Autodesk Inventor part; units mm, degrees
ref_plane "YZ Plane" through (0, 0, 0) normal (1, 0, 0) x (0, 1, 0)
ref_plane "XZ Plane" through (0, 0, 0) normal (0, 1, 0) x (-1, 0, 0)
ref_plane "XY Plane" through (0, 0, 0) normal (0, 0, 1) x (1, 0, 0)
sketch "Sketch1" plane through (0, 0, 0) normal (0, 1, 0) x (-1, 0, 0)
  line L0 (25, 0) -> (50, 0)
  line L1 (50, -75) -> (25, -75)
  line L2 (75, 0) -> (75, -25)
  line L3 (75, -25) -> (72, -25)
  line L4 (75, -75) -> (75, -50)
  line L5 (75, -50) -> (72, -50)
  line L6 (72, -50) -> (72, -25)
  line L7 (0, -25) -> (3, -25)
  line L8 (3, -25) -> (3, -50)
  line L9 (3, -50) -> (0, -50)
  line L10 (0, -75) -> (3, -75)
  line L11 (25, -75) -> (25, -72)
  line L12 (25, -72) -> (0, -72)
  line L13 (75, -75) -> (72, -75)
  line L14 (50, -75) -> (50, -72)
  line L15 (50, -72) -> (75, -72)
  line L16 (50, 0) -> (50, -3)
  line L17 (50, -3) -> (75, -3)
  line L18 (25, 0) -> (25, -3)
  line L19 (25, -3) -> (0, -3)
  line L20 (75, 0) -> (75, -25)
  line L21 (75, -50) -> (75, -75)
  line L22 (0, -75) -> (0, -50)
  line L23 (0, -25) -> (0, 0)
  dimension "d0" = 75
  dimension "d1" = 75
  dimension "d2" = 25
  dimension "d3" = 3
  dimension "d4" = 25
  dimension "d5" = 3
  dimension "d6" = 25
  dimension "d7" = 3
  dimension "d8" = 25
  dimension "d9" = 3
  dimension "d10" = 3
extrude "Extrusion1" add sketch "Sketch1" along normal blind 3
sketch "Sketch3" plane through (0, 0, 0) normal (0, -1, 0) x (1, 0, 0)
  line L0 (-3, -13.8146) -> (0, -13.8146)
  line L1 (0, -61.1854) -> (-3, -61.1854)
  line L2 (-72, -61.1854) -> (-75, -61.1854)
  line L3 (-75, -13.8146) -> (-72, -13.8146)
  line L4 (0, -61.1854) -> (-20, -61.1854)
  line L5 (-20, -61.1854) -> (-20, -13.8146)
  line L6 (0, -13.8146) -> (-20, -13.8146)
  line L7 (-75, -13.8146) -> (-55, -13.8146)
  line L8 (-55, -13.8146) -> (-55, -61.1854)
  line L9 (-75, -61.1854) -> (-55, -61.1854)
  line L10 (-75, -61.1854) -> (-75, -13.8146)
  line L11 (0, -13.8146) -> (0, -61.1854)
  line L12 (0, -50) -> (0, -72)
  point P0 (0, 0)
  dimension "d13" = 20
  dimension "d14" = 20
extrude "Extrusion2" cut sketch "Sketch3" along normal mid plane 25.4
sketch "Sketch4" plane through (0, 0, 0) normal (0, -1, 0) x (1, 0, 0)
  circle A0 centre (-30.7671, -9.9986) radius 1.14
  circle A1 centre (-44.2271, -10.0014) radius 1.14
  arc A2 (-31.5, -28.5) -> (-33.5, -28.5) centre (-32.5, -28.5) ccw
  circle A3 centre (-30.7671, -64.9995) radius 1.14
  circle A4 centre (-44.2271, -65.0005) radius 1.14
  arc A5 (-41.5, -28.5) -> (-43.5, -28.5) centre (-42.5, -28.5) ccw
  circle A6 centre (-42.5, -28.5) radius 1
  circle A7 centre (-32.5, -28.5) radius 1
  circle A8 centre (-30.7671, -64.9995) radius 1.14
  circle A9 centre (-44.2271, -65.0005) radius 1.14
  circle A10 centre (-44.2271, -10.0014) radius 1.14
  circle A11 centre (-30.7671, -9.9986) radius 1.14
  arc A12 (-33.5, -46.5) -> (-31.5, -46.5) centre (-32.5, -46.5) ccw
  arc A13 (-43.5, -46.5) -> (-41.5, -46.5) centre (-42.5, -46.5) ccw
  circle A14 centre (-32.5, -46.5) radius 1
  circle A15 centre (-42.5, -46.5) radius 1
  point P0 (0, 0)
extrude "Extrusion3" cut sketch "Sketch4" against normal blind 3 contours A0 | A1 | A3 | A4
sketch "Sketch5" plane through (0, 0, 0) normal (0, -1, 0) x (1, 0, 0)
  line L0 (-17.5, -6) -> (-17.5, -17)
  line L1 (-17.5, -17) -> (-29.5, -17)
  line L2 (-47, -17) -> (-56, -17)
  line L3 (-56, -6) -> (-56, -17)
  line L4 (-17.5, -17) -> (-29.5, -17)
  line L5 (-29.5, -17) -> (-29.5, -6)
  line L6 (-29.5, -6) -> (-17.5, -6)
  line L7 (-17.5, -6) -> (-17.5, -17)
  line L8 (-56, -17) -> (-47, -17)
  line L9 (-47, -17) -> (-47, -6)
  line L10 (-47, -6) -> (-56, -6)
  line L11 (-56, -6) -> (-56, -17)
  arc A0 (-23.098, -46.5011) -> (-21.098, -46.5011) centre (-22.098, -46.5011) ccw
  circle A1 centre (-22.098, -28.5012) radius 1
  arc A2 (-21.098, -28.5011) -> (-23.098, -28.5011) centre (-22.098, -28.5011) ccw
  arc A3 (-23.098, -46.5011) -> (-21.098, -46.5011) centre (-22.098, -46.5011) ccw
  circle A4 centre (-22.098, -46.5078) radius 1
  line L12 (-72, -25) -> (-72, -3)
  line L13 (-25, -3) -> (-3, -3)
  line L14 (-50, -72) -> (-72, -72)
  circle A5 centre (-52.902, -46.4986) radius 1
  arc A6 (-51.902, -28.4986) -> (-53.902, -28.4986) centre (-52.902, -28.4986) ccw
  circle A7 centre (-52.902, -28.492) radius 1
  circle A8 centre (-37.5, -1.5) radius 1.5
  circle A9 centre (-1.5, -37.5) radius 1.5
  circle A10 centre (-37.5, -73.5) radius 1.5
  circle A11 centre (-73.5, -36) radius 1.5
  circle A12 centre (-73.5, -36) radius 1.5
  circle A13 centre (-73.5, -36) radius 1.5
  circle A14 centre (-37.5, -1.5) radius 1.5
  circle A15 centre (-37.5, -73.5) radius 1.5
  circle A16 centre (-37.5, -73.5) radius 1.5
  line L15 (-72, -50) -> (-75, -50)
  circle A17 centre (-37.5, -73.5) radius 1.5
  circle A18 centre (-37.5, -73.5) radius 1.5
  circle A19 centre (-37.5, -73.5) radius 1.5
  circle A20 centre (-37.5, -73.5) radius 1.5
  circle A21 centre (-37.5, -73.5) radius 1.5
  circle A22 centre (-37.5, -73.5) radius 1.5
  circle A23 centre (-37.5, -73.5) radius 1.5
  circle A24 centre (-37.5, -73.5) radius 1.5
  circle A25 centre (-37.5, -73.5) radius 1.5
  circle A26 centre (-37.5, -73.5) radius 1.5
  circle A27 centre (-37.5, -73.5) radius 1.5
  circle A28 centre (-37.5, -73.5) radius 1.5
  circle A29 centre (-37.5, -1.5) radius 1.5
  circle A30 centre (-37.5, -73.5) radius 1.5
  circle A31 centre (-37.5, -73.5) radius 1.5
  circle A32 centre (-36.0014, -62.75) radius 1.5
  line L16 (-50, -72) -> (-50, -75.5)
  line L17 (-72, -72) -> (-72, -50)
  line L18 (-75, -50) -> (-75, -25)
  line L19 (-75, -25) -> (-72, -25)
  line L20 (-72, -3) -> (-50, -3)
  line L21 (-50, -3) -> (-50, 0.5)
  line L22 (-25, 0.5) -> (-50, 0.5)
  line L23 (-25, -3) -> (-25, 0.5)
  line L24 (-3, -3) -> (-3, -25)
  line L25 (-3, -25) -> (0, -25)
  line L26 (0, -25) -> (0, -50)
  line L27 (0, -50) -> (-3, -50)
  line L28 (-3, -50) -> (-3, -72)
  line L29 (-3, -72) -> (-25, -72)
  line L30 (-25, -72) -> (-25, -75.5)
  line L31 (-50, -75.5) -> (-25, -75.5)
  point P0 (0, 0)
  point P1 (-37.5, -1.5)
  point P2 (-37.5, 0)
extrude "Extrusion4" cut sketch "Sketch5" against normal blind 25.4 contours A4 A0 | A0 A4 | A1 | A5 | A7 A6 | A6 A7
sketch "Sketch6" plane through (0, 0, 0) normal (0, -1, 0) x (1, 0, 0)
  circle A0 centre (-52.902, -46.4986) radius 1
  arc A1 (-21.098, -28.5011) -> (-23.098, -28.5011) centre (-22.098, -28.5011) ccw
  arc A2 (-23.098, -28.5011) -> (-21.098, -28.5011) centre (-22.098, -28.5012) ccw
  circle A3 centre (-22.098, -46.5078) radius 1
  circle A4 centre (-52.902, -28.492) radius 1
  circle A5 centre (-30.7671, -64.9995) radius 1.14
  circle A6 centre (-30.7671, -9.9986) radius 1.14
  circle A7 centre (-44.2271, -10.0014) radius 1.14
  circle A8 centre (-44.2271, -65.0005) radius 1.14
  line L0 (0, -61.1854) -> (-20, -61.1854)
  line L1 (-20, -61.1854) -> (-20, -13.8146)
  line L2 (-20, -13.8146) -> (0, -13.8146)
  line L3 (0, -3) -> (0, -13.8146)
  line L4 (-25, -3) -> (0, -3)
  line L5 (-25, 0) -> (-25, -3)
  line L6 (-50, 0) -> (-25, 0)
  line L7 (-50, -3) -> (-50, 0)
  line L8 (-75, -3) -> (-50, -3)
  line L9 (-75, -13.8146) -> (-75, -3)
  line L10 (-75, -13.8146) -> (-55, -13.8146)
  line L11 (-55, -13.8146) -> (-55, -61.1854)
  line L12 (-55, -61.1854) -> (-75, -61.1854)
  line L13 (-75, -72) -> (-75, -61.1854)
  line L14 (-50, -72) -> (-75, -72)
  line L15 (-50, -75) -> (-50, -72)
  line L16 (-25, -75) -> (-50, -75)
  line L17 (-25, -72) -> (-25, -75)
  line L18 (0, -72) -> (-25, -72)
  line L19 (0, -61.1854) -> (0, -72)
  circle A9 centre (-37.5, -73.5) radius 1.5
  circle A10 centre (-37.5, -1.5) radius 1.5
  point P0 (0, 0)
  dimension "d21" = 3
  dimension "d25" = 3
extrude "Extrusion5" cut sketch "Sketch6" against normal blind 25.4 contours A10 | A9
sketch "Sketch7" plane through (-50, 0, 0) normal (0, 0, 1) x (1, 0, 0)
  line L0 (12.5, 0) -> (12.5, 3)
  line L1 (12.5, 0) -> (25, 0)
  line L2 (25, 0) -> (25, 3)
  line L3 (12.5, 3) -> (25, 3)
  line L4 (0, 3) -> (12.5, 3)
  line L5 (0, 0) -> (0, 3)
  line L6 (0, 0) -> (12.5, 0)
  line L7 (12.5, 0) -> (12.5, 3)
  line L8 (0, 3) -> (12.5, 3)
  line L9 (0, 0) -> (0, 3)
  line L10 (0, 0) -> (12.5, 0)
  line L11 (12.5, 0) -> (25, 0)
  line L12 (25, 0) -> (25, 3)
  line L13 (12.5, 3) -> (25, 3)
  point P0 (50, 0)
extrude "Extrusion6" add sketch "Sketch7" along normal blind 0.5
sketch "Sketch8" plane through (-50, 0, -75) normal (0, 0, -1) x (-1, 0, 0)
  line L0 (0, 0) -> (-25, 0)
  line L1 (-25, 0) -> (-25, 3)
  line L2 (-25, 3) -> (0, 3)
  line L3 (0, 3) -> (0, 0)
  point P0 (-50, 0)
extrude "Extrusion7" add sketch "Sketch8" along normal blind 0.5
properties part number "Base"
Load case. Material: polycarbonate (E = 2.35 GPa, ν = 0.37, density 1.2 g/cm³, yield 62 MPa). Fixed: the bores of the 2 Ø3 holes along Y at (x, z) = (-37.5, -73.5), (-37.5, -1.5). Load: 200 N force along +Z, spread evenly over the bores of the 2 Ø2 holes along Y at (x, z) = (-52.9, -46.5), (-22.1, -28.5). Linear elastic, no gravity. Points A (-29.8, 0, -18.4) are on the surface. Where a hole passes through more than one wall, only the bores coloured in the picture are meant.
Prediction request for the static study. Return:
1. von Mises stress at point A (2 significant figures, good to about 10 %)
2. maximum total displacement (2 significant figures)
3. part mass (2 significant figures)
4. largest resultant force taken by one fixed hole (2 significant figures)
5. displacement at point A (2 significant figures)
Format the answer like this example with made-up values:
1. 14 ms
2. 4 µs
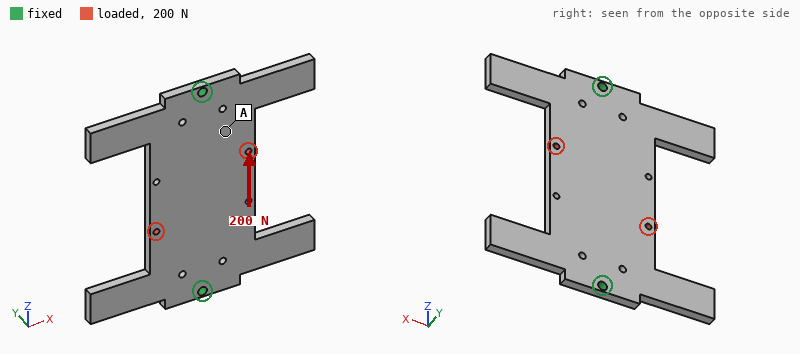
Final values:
1. 1.1 MPa
2. 47 µm
3. 12 g
4. 100 N
5. 25 µm
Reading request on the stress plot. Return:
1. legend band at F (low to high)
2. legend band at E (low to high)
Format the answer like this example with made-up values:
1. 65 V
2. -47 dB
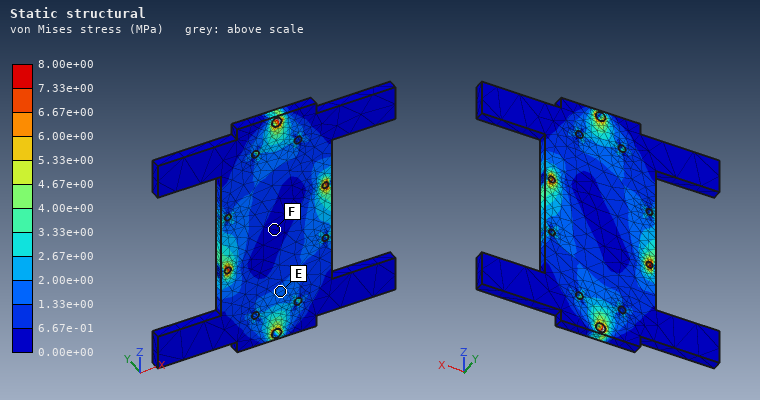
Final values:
1. 0.00e+00 to 6.67e-01 MPa
2. 1.33e+00 to 2.00e+00 MPa
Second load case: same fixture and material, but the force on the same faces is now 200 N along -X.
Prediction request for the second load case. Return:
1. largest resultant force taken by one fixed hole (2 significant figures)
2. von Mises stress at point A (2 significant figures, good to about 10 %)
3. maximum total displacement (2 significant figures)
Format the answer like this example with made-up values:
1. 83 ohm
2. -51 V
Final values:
1. 100 N
2. 2.7 MPa
3. 0.11 mm
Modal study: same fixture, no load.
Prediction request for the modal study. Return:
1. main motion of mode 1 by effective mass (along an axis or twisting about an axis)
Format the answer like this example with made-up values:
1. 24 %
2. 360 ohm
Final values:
1. twisting about Z
